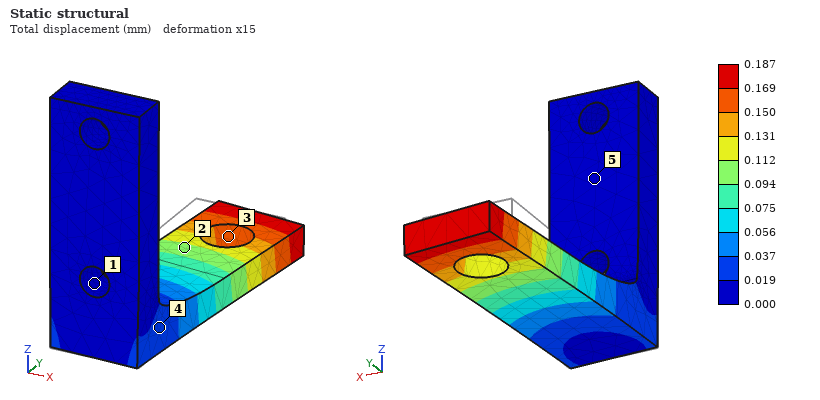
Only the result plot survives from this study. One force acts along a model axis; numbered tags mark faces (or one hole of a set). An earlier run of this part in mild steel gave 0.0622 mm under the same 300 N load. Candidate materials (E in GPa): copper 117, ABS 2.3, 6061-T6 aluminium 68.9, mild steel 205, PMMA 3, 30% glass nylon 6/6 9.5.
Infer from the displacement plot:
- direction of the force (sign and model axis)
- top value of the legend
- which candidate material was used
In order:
+X
0.187 mm
6061-T6 aluminium
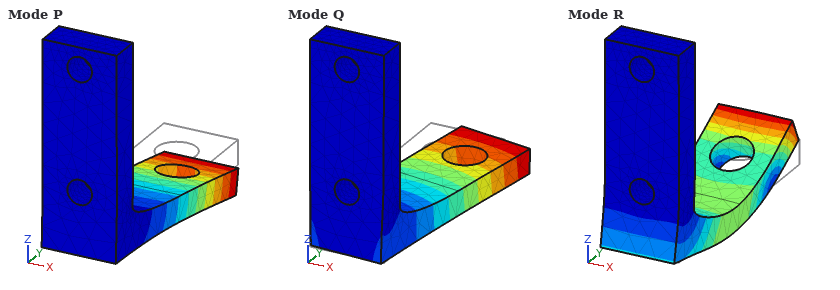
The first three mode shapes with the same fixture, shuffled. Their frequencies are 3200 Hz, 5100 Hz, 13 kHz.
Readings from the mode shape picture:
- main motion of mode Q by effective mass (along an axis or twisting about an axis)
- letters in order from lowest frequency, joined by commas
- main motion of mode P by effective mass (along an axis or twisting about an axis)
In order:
along X
P, Q, R
along Z
